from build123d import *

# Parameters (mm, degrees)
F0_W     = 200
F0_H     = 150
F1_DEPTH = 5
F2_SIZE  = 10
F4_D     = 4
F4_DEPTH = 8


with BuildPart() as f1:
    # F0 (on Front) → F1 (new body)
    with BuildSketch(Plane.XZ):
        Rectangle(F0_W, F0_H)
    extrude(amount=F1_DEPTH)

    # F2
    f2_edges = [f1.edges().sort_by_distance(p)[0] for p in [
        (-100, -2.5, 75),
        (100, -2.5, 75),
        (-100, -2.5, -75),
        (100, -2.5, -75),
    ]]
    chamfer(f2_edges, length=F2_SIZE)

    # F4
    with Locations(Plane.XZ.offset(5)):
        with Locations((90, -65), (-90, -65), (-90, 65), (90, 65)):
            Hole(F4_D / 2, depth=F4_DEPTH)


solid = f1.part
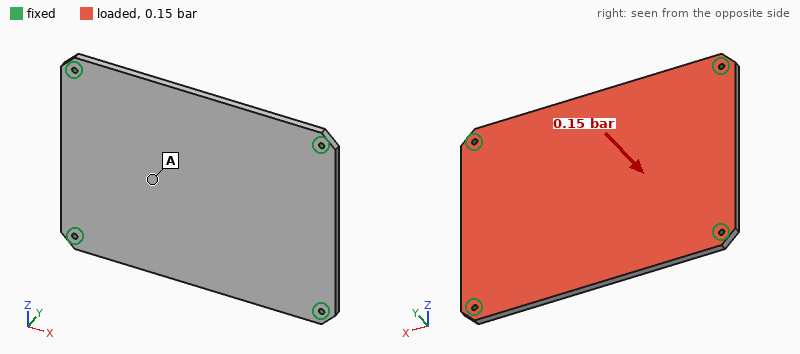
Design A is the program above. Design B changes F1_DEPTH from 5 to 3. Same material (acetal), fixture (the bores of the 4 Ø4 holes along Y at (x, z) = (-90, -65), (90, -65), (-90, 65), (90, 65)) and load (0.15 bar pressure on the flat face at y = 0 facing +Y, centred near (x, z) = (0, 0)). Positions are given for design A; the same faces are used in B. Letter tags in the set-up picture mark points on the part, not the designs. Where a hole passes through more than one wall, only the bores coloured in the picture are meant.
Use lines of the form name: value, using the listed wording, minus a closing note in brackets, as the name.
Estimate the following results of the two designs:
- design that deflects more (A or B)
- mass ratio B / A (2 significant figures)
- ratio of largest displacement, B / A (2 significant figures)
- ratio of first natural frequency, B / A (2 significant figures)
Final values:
design that deflects more: B
mass ratio B / A: 0.60
ratio of largest displacement, B / A: 4.4
ratio of first natural frequency, B / A: 0.62
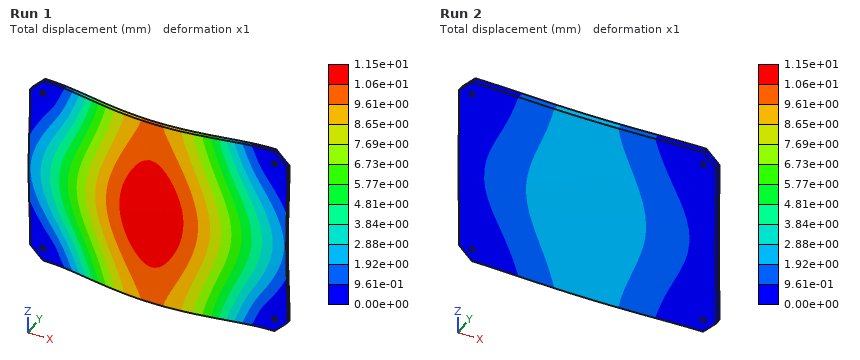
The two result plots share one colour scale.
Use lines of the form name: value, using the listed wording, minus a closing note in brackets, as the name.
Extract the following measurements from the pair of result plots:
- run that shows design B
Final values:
run that shows design B: Run 1
